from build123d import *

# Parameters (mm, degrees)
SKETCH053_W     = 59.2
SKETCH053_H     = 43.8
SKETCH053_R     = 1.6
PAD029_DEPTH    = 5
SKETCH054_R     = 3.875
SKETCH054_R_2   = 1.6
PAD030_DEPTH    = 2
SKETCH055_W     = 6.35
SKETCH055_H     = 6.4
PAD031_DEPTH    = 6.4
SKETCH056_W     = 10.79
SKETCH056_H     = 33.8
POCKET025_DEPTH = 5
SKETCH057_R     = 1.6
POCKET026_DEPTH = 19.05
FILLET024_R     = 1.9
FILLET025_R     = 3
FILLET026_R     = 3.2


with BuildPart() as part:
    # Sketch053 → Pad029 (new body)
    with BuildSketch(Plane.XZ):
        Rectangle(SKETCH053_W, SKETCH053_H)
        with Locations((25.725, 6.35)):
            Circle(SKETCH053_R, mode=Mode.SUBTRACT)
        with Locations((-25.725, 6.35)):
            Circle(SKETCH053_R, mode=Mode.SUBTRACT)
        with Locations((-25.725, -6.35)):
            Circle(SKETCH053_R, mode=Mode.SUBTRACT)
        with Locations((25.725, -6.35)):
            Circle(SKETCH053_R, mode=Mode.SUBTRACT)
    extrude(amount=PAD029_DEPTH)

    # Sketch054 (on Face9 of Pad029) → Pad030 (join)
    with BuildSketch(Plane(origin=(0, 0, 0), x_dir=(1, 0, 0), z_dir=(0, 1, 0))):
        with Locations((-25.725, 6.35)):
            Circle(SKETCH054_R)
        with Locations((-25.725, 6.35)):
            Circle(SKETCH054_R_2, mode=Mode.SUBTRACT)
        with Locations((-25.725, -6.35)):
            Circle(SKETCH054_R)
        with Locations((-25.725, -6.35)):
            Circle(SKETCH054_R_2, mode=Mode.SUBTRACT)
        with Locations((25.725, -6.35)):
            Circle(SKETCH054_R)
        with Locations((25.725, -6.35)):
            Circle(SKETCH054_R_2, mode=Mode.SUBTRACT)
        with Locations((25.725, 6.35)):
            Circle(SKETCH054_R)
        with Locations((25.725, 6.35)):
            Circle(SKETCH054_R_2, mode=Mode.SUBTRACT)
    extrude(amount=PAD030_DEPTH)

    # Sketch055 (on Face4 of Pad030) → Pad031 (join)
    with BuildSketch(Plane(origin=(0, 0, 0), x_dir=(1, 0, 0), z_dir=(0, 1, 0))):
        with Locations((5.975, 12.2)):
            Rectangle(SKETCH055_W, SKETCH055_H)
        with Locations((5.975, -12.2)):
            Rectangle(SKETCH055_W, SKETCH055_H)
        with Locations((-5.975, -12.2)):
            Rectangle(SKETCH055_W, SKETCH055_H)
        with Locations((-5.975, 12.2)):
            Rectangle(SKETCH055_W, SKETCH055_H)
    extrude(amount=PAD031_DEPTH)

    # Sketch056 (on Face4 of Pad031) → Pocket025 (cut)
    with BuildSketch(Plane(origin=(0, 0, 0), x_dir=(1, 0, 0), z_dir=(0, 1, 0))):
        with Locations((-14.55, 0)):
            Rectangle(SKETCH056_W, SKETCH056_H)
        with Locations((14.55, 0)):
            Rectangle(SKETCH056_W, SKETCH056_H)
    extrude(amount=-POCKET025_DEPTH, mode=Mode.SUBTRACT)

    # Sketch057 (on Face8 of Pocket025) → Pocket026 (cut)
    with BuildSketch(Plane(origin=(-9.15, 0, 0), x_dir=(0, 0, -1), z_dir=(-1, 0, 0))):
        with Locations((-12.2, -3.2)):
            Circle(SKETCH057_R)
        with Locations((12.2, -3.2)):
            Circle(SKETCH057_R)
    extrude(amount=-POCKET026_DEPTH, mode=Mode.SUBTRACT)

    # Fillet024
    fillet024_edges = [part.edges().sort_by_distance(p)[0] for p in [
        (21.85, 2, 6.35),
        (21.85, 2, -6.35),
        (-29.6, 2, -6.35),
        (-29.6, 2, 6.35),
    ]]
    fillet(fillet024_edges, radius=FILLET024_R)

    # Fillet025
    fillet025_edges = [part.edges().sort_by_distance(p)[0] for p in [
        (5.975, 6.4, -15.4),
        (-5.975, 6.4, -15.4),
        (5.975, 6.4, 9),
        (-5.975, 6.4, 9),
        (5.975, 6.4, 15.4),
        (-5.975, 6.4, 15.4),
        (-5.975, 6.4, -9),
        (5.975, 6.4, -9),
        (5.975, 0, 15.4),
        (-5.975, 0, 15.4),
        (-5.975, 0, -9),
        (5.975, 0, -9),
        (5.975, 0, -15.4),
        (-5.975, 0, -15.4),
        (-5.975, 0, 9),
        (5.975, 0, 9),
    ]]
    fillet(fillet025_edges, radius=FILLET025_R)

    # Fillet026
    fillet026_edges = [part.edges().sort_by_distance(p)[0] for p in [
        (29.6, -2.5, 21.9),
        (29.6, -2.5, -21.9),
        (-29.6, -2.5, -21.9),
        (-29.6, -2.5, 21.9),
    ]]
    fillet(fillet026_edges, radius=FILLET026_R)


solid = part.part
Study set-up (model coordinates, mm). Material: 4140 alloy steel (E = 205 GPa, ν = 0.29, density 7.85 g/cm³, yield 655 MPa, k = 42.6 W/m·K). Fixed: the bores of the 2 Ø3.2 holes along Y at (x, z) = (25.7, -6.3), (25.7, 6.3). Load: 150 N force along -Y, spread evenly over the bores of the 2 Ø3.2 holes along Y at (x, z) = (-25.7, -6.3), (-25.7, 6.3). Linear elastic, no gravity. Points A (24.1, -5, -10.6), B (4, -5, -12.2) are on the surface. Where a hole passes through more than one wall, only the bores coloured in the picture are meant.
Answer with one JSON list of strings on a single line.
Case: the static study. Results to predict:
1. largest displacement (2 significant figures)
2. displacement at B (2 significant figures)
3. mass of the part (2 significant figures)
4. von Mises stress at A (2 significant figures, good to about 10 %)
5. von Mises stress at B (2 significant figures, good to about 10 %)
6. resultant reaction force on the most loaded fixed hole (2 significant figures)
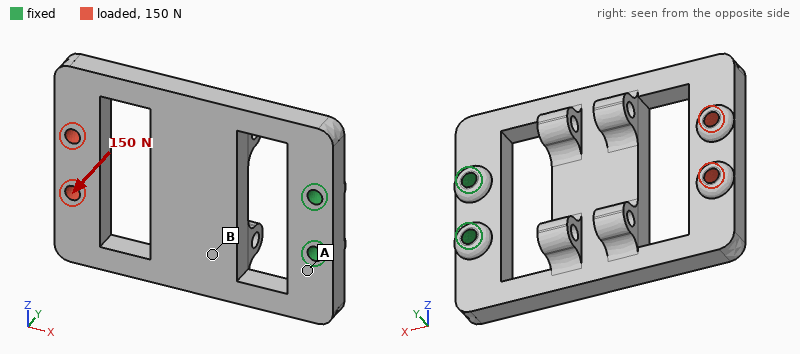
["0.36 mm", "0.093 mm", "80 g", "92 MPa", "22 MPa", "76 N"]
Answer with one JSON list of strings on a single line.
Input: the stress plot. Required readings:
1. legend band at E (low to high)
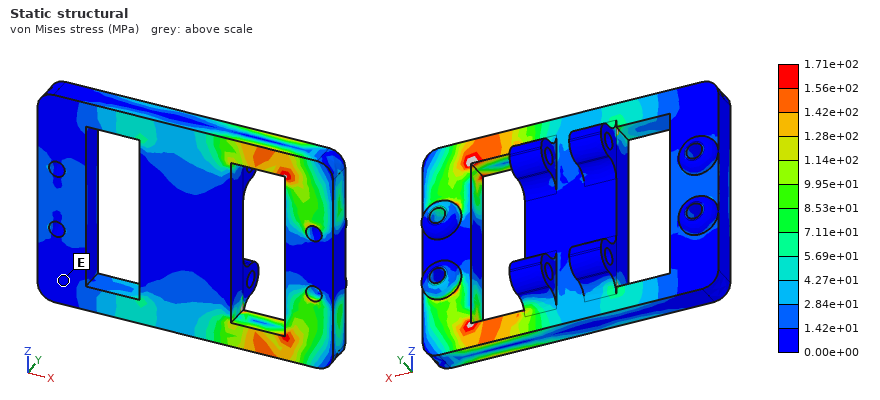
["0.00e+00 to 1.42e+01 MPa"]
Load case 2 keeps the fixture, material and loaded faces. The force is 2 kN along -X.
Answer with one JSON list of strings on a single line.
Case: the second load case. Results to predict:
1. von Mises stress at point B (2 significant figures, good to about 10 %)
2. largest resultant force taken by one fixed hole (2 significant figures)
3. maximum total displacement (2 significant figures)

["15 MPa", "1.2 kN", "0.14 mm"]
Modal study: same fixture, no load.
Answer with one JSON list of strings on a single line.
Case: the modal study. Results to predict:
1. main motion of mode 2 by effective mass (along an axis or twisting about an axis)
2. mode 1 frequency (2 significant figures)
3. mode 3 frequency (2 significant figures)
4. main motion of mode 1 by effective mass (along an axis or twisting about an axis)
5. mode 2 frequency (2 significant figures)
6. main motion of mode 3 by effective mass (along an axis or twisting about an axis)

["along Z", "700 Hz", "2700 Hz", "along Y", "2400 Hz", "twisting about X"]
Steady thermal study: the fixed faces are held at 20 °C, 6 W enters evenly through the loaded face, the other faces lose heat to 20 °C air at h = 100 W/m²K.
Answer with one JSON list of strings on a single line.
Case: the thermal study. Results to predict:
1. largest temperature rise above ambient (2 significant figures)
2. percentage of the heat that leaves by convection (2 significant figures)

["34 K", "95 %"]
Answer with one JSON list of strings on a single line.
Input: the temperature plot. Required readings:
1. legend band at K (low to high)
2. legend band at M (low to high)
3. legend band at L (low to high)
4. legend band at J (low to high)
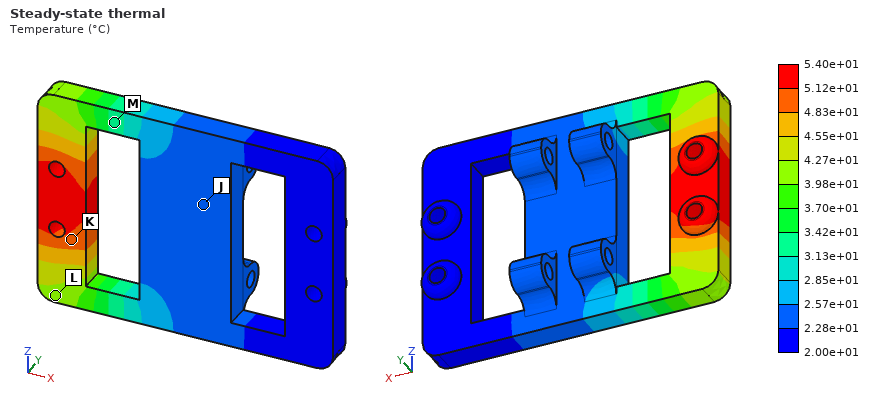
["4.83e+01 to 5.12e+01 °C", "3.13e+01 to 3.42e+01 °C", "3.98e+01 to 4.27e+01 °C", "2.28e+01 to 2.57e+01 °C"]
